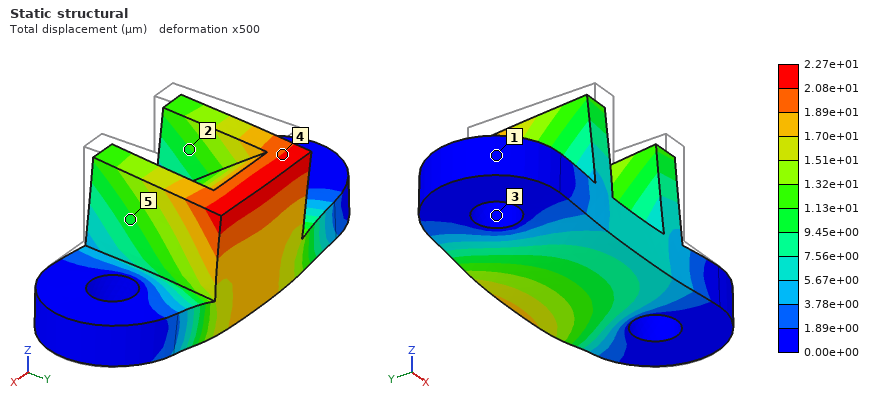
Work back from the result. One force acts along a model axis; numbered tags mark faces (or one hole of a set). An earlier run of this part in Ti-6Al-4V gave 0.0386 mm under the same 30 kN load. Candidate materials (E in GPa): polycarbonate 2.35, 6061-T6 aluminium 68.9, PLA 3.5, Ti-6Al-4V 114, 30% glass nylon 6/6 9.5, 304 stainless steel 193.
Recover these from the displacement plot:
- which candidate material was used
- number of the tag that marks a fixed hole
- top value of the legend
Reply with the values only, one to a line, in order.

304 stainless steel
3
2.27e+01 µm
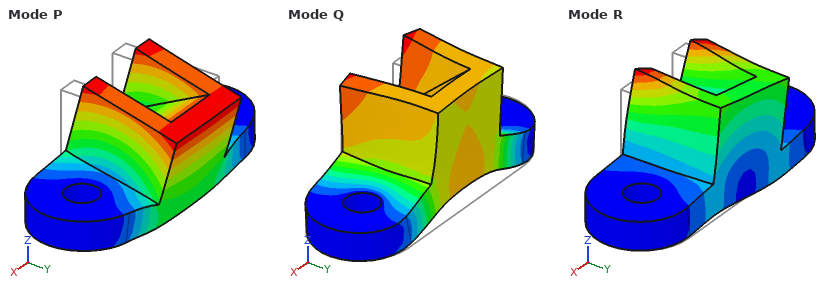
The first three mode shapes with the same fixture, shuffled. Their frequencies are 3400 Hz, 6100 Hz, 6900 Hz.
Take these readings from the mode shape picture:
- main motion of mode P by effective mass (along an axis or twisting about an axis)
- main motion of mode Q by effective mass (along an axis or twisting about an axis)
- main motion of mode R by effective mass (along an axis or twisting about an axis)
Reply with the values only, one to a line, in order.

along Y
along Z
along X
